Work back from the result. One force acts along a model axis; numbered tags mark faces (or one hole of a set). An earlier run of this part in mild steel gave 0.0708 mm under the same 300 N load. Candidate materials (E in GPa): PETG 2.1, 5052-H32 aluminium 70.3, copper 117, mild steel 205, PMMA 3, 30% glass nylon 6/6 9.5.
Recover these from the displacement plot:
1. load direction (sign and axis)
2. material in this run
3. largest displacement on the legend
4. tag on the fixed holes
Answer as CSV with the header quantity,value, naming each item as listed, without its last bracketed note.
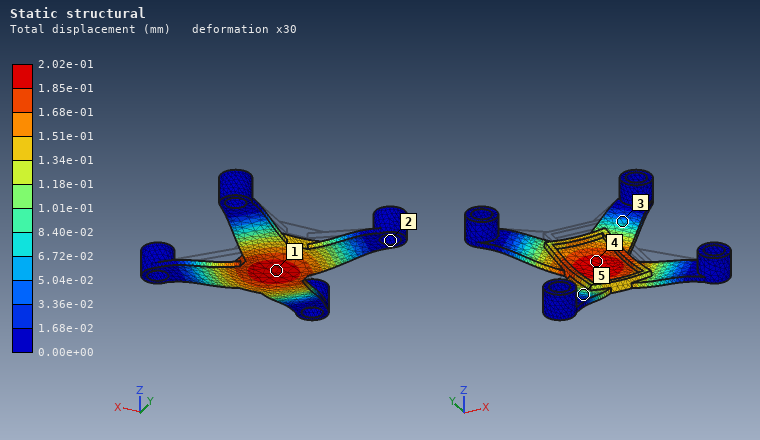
quantity,value
load direction,-Z
material in this run,5052-H32 aluminium
largest displacement on the legend,2.02e-01 mm
tag on the fixed holes,2
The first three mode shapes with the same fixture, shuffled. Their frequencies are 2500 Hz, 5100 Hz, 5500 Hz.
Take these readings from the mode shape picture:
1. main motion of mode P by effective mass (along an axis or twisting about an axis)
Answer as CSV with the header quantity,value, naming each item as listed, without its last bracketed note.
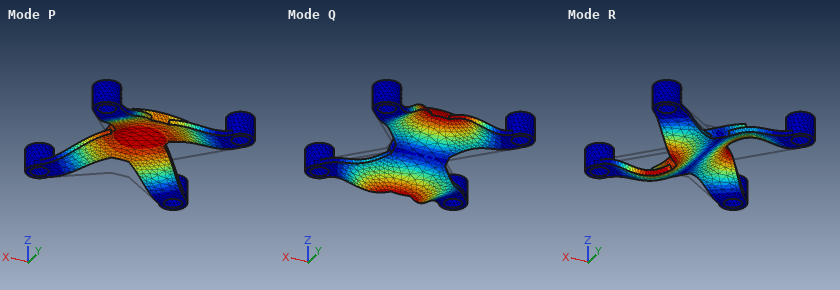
quantity,value
main motion of mode P by effective mass,along Z
